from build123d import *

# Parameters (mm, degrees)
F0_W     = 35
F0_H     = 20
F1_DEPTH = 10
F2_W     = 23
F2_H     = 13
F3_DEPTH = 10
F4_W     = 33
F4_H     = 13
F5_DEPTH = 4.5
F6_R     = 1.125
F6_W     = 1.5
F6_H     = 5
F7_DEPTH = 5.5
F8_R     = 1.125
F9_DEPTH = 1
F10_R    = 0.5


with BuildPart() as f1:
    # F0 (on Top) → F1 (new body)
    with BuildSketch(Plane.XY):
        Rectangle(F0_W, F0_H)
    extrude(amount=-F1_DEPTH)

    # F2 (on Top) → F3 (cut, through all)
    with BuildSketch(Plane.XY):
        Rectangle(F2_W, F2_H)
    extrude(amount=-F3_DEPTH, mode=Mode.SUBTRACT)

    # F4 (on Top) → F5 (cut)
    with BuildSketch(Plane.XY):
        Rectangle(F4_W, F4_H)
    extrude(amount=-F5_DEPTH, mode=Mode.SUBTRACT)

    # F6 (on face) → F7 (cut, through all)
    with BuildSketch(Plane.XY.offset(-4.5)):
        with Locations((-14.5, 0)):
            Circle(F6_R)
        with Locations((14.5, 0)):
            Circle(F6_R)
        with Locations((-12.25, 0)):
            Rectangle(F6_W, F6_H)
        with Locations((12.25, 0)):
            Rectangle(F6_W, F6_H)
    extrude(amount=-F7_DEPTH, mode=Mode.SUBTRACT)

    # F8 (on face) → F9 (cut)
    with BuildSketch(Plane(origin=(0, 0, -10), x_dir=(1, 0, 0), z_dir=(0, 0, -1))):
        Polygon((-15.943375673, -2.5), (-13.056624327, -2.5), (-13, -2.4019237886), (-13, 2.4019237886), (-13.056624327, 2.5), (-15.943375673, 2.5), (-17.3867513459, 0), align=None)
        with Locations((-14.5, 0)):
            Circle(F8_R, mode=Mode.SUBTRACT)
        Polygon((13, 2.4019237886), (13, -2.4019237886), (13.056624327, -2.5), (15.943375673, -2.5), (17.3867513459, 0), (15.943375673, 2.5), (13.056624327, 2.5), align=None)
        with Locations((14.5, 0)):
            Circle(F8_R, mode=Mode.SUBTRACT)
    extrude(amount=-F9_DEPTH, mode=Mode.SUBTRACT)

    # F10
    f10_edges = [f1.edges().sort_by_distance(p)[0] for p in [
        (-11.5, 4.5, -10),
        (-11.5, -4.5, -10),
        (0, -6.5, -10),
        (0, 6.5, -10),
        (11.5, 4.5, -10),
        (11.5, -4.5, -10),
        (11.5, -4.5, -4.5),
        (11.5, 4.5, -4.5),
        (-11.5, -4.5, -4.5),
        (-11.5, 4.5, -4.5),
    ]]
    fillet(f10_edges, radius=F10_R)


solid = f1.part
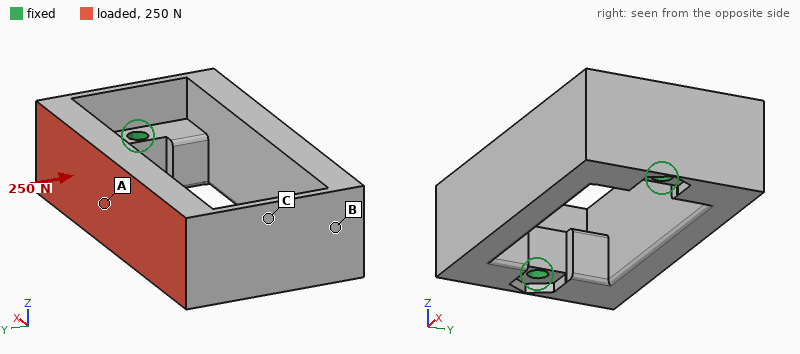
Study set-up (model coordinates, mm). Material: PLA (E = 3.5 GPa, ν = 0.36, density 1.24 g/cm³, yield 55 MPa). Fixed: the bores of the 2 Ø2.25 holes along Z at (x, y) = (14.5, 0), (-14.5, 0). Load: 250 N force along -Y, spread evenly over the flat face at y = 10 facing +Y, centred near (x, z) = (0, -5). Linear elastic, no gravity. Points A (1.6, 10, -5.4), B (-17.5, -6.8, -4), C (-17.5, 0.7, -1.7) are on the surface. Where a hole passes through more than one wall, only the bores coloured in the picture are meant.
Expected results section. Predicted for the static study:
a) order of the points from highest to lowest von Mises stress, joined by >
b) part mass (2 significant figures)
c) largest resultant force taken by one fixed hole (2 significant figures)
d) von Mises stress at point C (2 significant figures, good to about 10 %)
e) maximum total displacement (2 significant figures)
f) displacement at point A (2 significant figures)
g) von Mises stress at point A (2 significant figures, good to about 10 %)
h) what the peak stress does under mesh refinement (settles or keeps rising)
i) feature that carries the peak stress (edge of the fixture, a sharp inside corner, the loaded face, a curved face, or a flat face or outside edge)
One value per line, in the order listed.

A > C > B
4.0 g
150 N
4.9 MPa
0.22 mm
0.16 mm
14 MPa
keeps rising
a sharp inside corner
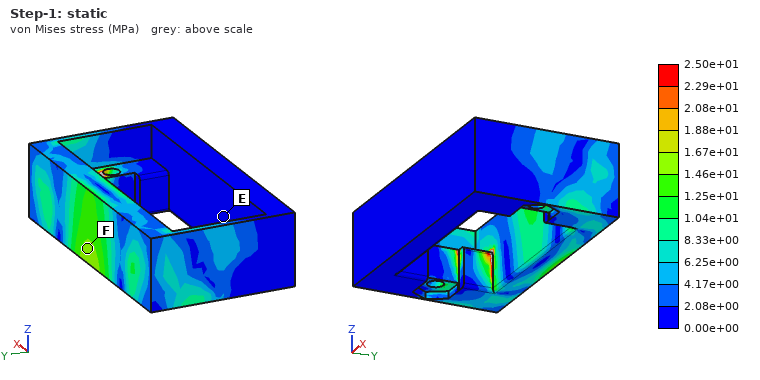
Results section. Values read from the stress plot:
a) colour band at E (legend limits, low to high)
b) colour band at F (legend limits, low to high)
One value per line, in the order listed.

0.00e+00 to 2.08e+00 MPa
1.46e+01 to 1.67e+01 MPa
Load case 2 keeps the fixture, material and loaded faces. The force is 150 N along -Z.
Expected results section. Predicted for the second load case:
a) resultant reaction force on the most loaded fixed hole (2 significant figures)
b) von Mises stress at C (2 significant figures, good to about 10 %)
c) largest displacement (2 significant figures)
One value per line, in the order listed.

75 N
10 MPa
0.21 mm
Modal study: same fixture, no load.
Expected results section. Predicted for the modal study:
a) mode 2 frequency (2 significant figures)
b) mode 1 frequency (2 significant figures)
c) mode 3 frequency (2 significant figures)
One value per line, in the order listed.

4900 Hz
4100 Hz
5100 Hz
